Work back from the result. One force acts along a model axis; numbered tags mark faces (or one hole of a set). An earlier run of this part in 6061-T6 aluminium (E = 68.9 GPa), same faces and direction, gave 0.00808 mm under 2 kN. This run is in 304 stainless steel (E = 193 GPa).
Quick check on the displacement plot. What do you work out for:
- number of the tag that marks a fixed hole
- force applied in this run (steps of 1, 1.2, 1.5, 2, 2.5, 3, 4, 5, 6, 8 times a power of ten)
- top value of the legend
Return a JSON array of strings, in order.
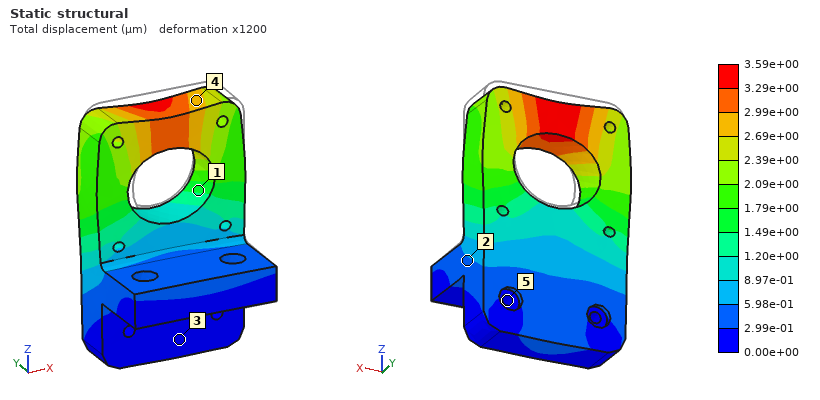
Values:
["5", "2.5 kN", "3.59e+00 µm"]
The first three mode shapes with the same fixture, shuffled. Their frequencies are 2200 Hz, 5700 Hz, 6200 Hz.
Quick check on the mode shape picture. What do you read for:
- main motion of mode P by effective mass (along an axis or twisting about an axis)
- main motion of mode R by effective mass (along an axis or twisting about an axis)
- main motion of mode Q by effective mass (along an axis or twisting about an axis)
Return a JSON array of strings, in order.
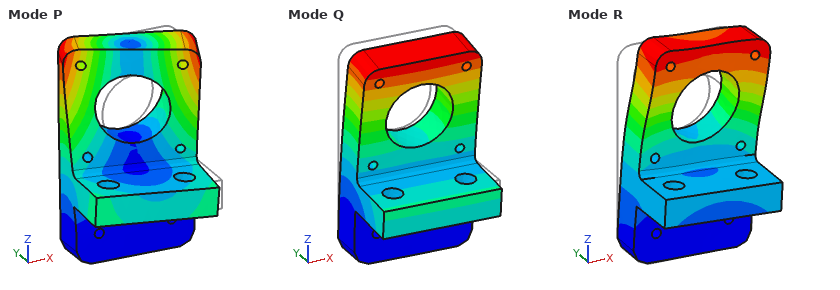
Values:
["twisting about Z", "along X", "along Y"]
